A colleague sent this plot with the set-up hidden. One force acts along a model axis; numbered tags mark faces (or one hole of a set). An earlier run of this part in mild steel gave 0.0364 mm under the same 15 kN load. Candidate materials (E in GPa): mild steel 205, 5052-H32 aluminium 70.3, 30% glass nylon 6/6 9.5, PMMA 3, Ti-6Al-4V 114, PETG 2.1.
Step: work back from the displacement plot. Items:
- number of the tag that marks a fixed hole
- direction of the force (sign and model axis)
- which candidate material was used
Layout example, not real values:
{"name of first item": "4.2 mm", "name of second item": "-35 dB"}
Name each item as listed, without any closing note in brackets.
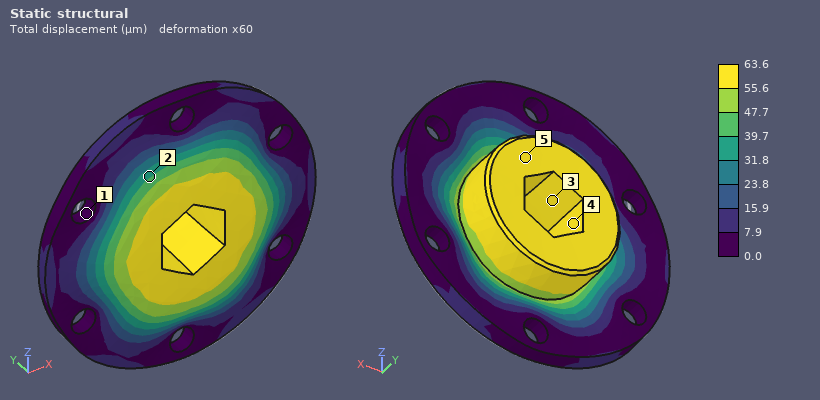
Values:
{"number of the tag that marks a fixed hole": "1", "direction of the force": "-Y", "which candidate material was used": "Ti-6Al-4V"}
